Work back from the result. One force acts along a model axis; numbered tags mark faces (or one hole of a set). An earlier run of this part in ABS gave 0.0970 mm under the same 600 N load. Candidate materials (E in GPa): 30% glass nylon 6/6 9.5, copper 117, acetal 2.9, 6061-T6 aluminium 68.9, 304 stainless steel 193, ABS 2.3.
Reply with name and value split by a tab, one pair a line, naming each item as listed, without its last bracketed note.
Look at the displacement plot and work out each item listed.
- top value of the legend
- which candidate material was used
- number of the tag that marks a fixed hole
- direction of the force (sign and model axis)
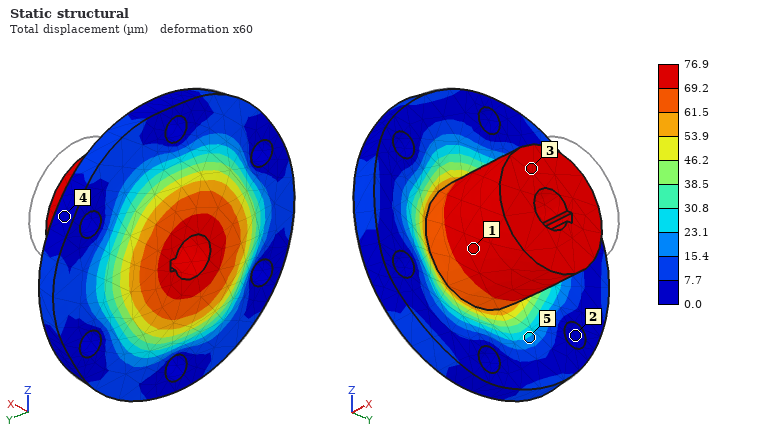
top value of the legend	76.9 µm
which candidate material was used	acetal
number of the tag that marks a fixed hole	2
direction of the force	-X
